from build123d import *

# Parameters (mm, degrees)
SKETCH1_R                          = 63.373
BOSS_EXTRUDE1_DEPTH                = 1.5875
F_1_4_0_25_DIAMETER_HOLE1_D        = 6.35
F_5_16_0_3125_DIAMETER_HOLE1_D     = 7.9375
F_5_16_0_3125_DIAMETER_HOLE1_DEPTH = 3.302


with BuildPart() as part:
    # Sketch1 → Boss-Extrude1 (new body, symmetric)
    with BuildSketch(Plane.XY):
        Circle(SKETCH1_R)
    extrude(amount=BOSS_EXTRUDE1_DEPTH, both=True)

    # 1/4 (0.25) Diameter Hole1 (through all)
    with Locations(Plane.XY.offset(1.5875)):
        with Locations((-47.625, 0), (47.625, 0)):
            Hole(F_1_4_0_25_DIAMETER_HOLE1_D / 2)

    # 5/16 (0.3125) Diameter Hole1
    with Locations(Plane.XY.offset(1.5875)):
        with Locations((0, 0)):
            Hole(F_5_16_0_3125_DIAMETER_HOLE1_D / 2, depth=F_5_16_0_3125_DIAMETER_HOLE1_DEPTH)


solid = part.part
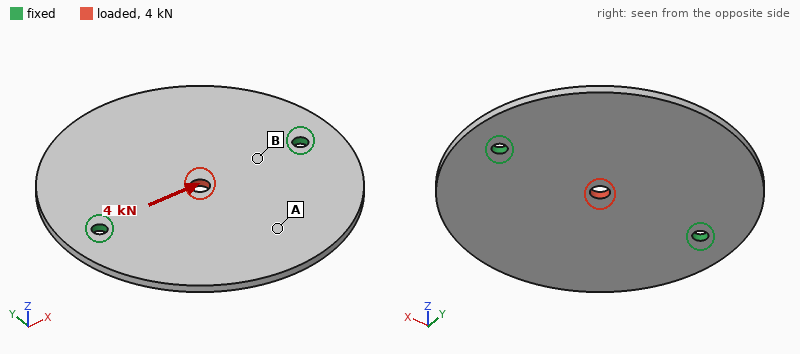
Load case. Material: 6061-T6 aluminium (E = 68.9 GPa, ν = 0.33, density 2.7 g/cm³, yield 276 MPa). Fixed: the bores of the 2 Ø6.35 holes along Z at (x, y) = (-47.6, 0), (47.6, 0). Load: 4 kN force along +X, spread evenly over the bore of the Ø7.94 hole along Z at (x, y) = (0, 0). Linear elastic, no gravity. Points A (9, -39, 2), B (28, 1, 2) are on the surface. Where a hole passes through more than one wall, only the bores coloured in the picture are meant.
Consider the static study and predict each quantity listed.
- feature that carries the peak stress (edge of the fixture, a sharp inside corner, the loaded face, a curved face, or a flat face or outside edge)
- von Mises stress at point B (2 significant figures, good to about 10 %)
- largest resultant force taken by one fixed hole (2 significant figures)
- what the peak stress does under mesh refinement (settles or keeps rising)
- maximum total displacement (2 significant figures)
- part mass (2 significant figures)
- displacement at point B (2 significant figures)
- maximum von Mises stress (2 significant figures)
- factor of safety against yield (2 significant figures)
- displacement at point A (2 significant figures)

the loaded face
23 MPa
2.0 kN
settles
18 µm
110 g
7.1 µm
87 MPa
3.2
7.3 µm
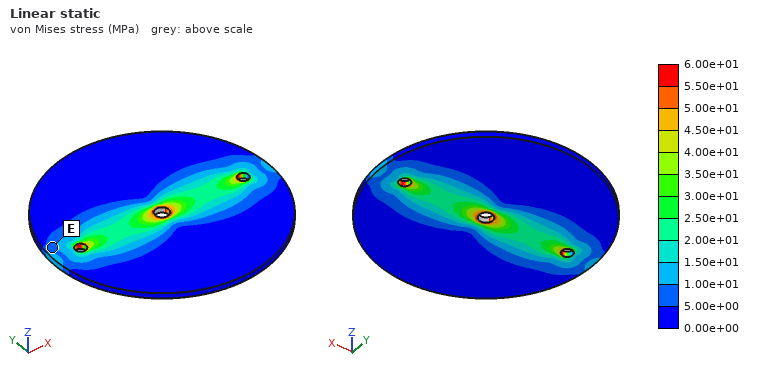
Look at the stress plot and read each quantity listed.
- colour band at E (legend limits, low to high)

5.00e+00 to 1.00e+01 MPa
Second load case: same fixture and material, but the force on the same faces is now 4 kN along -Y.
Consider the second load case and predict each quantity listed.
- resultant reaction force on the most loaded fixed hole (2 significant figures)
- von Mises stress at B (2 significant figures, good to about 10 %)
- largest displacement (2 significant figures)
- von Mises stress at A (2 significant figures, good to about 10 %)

2.0 kN
9.8 MPa
24 µm
9.7 MPa
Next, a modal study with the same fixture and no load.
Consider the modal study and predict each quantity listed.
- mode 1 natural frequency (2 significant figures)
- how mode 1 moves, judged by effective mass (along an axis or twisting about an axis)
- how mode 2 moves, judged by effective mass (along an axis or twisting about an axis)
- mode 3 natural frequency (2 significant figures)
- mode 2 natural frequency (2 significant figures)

600 Hz
twisting about X
along Z
1700 Hz
780 Hz
